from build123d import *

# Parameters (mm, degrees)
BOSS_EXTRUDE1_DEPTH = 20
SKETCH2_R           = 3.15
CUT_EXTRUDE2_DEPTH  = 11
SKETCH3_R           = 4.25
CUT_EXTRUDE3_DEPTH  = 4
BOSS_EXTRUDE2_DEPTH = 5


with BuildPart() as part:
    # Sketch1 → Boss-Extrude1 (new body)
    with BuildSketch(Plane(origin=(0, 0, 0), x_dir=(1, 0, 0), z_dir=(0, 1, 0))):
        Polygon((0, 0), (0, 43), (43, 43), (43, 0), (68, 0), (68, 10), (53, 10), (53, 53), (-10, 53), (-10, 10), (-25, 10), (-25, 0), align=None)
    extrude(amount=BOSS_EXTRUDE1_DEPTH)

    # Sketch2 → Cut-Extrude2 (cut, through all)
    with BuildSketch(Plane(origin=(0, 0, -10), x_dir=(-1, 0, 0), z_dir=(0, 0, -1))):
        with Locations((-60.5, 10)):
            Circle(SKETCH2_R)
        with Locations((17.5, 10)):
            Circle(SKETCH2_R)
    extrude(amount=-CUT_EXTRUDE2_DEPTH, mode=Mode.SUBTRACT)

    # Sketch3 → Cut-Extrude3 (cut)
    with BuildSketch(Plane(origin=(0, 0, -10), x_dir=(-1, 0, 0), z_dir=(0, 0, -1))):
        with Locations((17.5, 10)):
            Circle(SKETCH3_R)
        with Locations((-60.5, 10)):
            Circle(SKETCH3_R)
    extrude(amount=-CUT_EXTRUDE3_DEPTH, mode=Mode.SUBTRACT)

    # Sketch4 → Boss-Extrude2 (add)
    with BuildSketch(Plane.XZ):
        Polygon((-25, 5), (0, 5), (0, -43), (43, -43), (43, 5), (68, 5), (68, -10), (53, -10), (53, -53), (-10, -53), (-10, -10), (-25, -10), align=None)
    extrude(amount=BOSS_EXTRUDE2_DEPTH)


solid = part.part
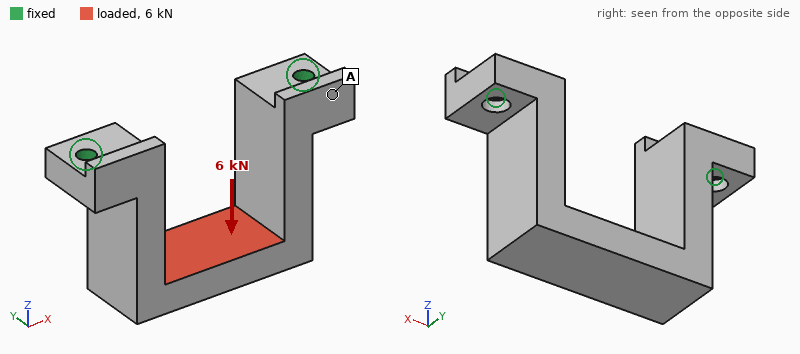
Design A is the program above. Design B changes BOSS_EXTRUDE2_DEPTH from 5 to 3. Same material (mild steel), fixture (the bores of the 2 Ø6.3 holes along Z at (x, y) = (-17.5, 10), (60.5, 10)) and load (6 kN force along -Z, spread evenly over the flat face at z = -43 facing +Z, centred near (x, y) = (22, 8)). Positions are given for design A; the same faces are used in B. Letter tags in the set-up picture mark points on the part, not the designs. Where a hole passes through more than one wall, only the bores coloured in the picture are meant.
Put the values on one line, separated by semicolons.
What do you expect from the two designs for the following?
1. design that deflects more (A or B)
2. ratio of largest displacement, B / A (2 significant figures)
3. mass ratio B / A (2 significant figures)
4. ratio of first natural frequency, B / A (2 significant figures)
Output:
A; 0.92; 0.91; 1.0
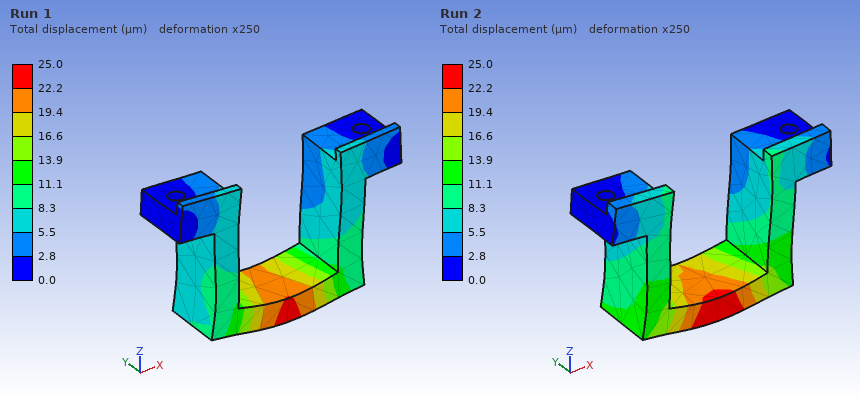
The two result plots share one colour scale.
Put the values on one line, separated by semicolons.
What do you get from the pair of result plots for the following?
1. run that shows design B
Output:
Run 1
